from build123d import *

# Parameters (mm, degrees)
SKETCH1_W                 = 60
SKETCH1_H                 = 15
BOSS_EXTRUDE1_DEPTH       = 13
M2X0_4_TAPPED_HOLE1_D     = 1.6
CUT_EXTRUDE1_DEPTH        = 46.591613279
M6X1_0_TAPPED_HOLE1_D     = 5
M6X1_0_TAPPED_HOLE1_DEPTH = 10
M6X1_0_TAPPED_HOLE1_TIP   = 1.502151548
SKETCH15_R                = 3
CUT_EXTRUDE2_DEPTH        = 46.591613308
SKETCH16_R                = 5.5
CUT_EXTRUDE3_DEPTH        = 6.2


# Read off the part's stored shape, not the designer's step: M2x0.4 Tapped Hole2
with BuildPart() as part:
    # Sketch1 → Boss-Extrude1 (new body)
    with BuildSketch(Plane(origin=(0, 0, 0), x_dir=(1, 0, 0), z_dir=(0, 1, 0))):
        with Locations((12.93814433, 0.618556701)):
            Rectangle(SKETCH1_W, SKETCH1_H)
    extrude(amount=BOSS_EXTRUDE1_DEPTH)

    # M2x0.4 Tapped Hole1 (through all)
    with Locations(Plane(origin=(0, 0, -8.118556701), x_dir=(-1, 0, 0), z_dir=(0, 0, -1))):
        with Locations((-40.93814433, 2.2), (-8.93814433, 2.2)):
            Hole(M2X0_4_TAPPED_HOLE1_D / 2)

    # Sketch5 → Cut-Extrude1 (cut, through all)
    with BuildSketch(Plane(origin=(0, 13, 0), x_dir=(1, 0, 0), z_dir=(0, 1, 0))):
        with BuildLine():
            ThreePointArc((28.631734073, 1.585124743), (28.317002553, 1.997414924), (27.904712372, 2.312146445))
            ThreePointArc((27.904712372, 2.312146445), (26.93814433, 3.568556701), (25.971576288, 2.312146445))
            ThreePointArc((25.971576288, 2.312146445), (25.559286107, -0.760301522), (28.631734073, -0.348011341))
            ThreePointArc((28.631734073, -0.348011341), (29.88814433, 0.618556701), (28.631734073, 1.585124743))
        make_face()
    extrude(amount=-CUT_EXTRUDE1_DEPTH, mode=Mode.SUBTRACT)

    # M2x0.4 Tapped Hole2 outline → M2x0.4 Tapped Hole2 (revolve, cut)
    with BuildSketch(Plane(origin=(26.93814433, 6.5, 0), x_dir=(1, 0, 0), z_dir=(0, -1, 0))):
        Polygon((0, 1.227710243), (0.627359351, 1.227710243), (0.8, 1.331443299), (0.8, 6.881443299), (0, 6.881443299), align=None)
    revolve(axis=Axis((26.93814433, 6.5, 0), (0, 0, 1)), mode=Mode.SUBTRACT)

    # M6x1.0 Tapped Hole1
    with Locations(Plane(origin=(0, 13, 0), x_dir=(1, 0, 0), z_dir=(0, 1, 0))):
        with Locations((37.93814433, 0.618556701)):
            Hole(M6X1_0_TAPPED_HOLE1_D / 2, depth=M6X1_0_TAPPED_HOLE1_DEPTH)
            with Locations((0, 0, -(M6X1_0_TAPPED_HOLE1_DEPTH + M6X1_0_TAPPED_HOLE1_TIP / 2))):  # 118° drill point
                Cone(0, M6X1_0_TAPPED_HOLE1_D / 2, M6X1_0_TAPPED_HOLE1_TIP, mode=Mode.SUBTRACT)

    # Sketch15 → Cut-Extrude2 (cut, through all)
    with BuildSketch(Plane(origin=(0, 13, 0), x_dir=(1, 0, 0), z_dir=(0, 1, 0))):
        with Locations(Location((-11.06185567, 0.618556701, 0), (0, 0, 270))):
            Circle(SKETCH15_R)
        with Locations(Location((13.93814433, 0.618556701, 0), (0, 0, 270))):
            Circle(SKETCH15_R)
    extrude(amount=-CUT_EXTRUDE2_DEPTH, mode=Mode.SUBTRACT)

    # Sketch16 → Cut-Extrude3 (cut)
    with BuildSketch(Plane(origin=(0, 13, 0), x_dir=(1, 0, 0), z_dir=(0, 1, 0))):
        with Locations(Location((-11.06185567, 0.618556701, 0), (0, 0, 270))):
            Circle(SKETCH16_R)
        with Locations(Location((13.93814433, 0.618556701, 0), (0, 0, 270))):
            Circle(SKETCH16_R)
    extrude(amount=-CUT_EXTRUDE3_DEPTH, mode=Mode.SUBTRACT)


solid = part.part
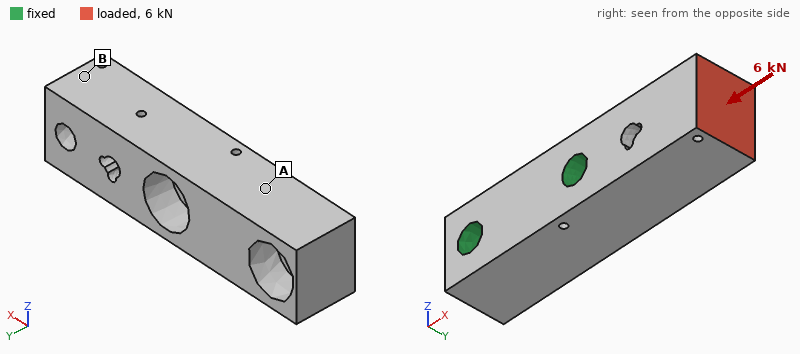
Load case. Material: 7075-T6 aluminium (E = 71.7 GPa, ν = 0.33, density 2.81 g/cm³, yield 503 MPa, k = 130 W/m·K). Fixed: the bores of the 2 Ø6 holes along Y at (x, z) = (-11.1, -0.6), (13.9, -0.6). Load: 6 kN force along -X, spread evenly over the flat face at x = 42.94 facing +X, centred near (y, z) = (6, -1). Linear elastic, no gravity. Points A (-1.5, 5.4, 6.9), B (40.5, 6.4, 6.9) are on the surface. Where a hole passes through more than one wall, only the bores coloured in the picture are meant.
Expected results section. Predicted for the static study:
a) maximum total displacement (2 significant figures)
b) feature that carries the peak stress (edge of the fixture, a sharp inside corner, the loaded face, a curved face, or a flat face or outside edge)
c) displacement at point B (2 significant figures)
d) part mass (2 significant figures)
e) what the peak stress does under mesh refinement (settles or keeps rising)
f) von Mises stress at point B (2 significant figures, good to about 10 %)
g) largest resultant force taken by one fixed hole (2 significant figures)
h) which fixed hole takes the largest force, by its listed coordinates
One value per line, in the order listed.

48 µm
a sharp inside corner
35 µm
27 g
keeps rising
25 MPa
5.1 kN
(13.9, -0.6)
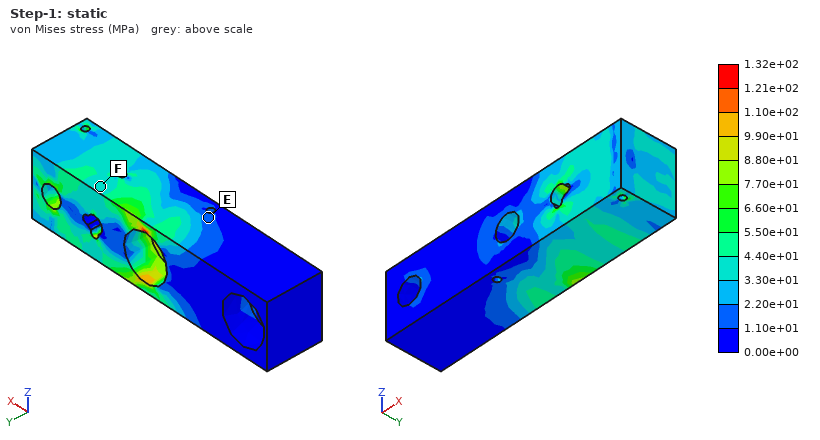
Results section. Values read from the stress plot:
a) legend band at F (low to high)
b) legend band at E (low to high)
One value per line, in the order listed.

3.30e+01 to 4.40e+01 MPa
1.10e+01 to 2.20e+01 MPa
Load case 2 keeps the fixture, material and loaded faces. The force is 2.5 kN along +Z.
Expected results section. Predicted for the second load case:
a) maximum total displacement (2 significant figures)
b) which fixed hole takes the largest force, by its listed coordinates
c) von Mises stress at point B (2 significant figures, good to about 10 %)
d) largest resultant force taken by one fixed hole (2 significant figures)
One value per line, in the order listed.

0.16 mm
(13.9, -0.6)
18 MPa
3.8 kN
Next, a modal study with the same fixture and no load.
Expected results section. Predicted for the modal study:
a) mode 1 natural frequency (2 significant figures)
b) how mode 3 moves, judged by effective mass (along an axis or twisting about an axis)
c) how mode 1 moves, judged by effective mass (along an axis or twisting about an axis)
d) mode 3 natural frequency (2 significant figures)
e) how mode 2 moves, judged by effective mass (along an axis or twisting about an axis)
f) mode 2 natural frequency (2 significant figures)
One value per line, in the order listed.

8400 Hz
twisting about X
along Y
19 kHz
along Z
9900 Hz
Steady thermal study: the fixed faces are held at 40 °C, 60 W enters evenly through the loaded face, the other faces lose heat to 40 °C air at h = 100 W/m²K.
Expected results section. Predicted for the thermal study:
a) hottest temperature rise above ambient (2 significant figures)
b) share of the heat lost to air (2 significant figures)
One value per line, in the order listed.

80 K
15 %
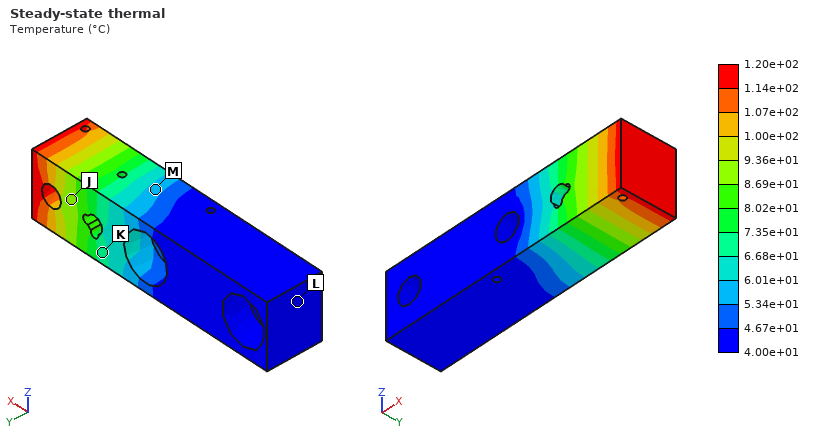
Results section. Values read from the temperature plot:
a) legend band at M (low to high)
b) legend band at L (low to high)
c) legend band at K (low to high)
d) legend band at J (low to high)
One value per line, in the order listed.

5.34e+01 to 6.01e+01 °C
4.00e+01 to 4.67e+01 °C
6.68e+01 to 7.35e+01 °C
8.69e+01 to 9.36e+01 °C
